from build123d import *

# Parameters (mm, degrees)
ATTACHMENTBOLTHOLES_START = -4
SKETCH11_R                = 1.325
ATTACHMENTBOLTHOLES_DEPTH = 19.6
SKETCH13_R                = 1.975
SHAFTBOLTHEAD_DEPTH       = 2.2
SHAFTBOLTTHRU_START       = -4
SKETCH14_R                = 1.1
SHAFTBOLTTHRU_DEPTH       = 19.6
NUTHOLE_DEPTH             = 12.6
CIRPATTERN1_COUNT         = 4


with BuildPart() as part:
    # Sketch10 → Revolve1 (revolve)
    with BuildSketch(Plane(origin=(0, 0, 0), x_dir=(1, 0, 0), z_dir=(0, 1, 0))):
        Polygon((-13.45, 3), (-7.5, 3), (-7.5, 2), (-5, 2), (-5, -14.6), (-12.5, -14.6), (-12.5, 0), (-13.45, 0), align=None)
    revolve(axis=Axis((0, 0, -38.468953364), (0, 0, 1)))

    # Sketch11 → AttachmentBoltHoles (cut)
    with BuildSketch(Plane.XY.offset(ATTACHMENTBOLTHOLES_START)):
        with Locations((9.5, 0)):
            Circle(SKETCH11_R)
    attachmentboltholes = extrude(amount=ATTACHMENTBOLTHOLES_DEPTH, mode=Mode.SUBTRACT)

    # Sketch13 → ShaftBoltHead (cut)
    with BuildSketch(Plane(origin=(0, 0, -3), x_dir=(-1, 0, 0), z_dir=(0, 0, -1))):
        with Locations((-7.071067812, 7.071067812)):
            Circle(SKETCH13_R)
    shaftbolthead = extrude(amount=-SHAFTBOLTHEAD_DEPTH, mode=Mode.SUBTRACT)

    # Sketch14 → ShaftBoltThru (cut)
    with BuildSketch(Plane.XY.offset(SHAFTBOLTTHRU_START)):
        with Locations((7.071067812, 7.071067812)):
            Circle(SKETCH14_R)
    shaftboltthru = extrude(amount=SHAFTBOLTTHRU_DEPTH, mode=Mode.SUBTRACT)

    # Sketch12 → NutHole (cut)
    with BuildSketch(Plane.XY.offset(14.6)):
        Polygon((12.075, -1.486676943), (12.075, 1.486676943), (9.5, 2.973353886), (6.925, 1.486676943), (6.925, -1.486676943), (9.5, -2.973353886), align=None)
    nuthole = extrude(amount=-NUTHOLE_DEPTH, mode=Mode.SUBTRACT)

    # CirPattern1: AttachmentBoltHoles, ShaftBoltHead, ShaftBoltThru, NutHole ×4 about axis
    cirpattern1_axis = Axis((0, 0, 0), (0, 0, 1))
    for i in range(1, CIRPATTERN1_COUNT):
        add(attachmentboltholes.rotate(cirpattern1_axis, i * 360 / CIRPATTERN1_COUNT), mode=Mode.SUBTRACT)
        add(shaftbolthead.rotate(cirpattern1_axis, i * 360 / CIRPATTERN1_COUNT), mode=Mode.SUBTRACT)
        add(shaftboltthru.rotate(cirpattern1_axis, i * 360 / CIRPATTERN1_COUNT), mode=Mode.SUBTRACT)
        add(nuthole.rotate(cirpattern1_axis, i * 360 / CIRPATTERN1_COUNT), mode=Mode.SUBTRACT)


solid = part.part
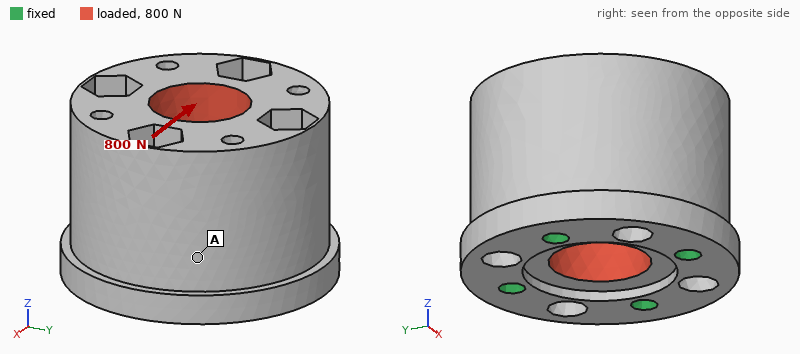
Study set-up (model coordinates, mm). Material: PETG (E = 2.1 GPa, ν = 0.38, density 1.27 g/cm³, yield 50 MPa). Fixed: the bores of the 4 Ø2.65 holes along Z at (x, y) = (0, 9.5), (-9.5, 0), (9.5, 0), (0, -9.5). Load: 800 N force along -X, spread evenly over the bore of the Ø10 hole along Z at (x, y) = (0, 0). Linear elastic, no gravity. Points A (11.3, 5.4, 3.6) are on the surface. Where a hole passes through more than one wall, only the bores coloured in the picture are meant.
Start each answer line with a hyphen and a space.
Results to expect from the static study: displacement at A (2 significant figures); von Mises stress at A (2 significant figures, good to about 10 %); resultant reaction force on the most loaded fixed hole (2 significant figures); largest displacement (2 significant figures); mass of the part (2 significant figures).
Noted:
- 42 µm
- 2.8 MPa
- 310 N
- 96 µm
- 7.3 g
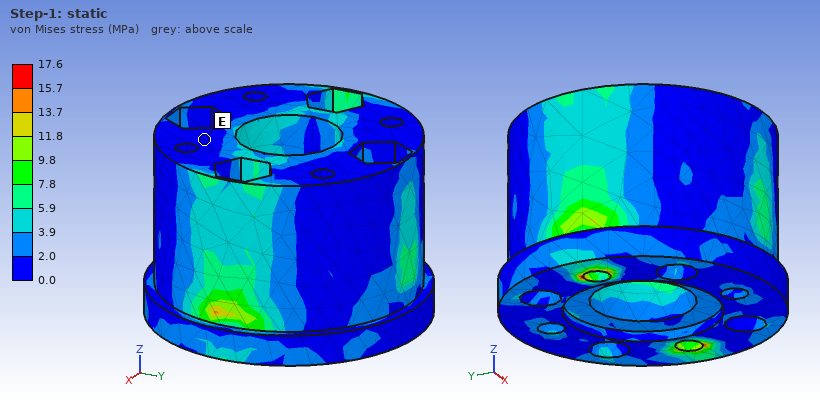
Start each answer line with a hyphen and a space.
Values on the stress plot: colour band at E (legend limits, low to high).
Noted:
- 0.0 to 2.0 MPa
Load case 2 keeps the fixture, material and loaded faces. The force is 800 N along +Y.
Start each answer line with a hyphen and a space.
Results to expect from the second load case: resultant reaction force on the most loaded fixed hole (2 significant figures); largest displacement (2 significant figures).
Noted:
- 310 N
- 96 µm
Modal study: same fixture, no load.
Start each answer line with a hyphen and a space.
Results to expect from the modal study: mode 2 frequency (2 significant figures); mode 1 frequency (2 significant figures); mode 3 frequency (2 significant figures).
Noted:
- 7100 Hz
- 7000 Hz
- 9200 Hz
